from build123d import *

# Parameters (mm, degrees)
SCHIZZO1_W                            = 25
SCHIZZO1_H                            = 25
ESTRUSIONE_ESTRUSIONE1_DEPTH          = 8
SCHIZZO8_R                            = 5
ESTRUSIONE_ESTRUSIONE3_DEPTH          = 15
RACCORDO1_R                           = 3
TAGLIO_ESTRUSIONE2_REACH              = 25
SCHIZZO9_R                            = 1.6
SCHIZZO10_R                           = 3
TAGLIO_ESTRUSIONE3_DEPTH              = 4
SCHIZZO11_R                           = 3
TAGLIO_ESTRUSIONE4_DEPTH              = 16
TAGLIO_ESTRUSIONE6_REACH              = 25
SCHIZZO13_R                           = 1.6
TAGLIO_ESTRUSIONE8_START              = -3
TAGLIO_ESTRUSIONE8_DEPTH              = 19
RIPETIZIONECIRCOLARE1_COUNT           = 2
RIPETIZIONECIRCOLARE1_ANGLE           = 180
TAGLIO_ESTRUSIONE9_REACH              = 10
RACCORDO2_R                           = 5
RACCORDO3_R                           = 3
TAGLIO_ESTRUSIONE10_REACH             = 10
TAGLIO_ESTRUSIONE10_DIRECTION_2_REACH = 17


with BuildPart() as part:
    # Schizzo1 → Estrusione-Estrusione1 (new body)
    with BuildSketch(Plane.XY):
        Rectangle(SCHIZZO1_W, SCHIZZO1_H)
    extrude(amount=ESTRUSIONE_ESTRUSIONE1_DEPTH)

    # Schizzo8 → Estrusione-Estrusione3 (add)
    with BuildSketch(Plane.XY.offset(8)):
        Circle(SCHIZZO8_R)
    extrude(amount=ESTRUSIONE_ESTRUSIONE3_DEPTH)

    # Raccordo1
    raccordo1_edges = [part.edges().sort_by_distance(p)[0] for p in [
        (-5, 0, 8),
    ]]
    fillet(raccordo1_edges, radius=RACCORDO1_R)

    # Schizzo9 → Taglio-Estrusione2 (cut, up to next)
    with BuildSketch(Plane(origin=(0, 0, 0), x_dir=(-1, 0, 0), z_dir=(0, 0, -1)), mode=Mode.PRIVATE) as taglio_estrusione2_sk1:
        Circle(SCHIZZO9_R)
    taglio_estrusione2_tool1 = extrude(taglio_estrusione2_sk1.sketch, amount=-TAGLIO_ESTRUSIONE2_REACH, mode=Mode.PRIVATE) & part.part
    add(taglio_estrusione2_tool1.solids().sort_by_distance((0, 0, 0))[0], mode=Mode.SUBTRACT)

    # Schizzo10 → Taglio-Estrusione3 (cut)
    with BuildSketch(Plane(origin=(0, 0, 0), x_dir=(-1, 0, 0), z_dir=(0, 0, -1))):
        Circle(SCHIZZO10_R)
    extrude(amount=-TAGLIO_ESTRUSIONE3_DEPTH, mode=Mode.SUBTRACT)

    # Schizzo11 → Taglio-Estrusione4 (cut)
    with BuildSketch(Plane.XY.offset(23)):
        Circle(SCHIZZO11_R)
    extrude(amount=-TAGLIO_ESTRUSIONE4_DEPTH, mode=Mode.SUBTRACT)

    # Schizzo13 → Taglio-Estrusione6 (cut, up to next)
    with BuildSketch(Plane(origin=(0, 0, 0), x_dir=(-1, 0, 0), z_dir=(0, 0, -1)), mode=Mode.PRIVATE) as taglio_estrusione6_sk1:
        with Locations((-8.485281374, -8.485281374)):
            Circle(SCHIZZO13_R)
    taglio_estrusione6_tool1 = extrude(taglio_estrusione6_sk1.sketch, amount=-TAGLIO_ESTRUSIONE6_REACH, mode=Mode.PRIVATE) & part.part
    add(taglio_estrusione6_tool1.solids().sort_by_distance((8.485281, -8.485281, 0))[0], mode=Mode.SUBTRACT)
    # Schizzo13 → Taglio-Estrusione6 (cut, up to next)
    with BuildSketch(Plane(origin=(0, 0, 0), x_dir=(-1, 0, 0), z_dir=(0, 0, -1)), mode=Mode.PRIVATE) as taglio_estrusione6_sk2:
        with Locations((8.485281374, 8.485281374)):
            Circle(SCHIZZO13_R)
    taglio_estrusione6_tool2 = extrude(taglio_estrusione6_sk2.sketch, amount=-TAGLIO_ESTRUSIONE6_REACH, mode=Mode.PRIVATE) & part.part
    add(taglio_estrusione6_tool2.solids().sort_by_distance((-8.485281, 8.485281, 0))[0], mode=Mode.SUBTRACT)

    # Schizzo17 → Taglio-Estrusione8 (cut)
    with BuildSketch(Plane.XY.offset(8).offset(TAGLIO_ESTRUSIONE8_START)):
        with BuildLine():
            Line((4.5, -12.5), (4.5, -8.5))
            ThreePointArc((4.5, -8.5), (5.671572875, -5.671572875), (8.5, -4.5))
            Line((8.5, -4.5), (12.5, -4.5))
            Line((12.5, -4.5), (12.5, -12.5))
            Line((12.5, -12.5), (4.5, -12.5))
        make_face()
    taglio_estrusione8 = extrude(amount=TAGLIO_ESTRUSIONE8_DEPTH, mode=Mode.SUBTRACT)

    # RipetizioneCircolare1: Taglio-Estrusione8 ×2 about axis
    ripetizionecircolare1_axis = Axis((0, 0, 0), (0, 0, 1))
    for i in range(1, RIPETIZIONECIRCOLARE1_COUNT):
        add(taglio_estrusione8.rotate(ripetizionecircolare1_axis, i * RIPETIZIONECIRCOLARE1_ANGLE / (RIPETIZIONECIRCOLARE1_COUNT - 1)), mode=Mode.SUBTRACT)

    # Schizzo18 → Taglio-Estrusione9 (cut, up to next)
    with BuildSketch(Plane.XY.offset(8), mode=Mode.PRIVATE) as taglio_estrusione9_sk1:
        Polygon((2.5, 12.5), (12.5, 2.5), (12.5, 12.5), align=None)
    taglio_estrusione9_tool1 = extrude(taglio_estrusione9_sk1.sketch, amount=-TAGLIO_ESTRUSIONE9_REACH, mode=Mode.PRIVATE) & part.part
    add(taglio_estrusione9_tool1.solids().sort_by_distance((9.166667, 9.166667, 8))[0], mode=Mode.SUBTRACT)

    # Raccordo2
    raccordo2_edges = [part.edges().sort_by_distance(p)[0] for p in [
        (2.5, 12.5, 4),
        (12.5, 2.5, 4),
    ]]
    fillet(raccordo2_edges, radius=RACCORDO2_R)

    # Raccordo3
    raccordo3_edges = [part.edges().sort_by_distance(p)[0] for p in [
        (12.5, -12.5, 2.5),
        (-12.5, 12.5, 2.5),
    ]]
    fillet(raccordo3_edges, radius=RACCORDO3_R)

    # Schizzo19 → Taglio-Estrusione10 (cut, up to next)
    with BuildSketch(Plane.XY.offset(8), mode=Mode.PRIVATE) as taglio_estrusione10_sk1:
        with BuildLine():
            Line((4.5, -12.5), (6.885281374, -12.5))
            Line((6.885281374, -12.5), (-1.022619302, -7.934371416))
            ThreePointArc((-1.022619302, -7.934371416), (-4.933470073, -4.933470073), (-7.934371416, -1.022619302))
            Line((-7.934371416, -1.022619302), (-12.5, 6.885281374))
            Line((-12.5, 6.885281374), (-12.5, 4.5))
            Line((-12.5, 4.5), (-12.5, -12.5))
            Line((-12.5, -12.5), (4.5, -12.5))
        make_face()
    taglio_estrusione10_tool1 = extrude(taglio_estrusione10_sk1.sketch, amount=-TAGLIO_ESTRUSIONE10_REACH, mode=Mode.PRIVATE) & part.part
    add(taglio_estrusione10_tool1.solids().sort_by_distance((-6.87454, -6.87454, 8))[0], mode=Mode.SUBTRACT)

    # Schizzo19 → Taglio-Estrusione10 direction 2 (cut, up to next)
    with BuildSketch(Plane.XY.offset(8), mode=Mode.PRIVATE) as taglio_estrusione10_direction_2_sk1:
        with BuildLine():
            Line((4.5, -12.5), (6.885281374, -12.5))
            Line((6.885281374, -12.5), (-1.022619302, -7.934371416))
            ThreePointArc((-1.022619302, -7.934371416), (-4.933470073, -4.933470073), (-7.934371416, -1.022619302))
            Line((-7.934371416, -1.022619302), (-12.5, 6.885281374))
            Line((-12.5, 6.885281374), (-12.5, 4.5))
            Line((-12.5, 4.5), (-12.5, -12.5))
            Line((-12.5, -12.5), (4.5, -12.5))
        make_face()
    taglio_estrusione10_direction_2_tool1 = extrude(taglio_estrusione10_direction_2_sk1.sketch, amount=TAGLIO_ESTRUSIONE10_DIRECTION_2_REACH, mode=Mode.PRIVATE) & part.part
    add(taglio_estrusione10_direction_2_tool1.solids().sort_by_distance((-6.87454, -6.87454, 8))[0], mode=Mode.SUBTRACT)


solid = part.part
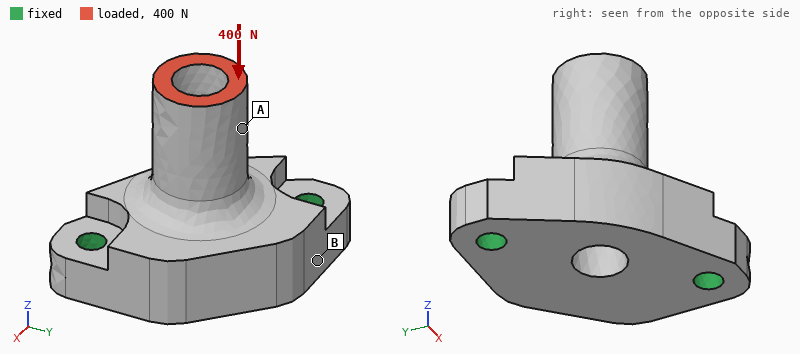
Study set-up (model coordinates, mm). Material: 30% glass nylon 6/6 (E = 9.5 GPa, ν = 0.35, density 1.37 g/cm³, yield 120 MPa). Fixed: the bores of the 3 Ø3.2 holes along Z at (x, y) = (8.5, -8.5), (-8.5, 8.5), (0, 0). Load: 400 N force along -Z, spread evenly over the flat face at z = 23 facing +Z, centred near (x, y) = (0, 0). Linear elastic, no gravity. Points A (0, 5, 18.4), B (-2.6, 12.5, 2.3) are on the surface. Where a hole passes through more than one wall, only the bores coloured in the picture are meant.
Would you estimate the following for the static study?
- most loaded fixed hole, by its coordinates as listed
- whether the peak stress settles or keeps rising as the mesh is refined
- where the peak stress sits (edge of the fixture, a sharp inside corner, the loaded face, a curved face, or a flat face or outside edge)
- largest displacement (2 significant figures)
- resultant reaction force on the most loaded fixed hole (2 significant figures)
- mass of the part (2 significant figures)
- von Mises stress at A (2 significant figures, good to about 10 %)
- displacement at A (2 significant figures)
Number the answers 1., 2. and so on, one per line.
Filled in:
1. (0, 0)
2. keeps rising
3. edge of the fixture
4. 17 µm
5. 240 N
6. 5.0 g
7. 7.9 MPa
8. 12 µm
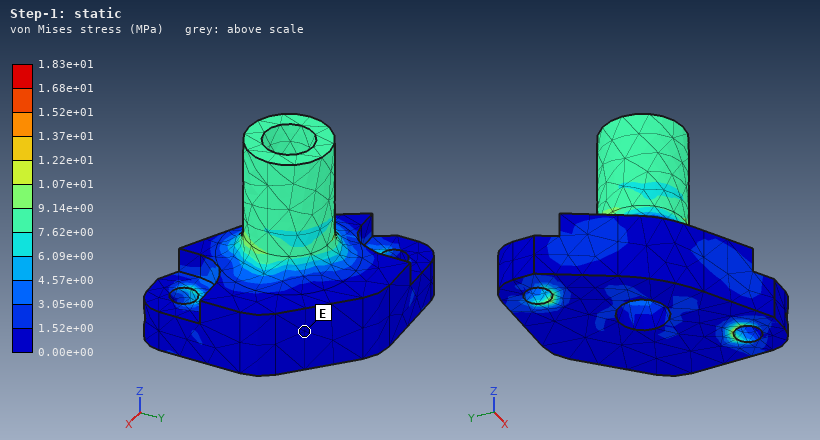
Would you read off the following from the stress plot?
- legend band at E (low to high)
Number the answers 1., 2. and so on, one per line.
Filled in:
1. 0.00e+00 to 1.52e+00 MPa
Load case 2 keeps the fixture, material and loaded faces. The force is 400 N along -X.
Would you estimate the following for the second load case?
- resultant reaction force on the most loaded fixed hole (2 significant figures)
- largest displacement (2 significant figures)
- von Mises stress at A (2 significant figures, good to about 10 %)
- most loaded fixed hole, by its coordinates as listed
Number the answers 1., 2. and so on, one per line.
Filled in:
1. 610 N
2. 0.26 mm
3. 22 MPa
4. (0, 0)
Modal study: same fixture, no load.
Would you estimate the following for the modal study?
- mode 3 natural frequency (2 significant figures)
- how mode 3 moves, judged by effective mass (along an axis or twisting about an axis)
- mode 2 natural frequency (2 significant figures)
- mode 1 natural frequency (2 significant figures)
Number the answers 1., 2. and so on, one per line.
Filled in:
1. 20 kHz
2. along Z
3. 13 kHz
4. 9200 Hz
